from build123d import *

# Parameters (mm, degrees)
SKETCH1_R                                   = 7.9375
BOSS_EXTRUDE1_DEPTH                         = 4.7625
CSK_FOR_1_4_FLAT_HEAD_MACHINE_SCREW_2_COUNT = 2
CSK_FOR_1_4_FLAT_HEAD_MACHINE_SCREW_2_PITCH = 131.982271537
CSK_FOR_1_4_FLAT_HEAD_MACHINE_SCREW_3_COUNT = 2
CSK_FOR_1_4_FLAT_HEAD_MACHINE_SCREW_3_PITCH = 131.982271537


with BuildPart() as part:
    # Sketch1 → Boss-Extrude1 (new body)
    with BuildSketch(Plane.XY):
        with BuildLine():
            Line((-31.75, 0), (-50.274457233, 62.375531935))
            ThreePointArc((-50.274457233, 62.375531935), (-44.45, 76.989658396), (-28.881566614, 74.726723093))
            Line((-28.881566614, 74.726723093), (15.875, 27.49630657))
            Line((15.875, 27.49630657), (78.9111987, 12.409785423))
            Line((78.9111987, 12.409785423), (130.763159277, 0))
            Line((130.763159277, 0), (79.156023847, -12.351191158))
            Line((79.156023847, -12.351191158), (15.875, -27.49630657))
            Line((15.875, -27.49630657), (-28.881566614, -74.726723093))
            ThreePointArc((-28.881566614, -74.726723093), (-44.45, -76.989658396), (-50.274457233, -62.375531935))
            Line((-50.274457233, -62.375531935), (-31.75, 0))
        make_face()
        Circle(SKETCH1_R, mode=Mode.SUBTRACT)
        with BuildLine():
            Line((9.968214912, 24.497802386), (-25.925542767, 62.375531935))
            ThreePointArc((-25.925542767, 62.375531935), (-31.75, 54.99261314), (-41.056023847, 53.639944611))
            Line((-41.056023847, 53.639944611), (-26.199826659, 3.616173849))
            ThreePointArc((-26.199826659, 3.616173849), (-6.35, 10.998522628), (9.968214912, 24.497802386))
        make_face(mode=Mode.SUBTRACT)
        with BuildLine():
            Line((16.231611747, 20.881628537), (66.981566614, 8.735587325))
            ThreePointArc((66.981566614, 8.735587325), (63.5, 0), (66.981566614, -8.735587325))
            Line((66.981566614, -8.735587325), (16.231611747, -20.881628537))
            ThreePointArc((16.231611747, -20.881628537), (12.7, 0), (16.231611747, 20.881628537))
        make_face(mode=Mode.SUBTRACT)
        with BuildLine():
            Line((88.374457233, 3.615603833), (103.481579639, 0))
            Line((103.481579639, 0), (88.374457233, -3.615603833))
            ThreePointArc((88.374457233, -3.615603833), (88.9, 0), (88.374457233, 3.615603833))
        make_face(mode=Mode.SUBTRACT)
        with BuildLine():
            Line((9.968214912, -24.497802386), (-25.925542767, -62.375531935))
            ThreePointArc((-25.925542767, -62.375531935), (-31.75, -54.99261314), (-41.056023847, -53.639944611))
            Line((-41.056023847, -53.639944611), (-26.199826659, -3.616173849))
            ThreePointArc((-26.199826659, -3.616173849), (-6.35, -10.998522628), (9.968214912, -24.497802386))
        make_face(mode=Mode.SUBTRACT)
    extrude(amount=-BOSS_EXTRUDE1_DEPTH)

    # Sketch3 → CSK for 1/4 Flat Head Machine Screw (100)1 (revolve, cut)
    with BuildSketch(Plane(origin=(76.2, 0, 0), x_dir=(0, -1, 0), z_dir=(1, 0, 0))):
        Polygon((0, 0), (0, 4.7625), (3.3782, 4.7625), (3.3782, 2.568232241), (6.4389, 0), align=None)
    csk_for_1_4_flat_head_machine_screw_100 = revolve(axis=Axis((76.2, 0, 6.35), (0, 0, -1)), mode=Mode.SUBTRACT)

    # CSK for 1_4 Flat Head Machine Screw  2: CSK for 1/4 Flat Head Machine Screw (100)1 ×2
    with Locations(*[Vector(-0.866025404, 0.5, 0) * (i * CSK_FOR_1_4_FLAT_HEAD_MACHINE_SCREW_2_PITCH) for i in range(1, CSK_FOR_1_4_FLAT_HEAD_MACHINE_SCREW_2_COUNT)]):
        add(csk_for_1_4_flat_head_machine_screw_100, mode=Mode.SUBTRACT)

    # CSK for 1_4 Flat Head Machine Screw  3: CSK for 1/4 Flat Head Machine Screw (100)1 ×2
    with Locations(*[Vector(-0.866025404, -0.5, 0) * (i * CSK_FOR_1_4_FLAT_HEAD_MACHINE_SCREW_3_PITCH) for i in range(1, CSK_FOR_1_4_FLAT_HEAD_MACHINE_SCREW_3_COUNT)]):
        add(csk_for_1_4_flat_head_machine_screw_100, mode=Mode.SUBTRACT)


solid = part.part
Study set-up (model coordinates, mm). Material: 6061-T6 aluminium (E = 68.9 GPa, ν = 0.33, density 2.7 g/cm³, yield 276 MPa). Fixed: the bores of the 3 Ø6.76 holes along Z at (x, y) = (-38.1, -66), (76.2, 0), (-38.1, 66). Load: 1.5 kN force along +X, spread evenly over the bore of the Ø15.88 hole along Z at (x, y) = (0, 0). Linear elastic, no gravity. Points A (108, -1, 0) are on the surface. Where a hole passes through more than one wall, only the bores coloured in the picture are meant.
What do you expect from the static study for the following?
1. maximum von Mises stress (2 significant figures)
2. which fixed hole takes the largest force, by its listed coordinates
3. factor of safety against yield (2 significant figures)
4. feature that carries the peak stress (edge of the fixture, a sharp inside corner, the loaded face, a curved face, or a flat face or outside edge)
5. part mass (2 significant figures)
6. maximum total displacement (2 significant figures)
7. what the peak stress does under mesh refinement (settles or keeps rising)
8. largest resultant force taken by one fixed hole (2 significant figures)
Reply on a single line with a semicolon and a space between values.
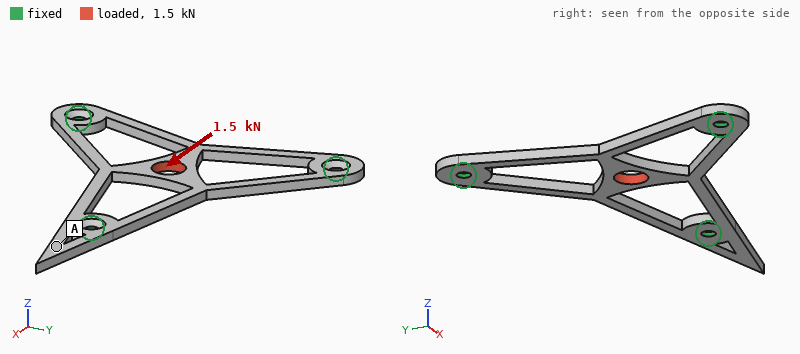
91 MPa; (76.2, 0); 3.0; a curved face; 61 g; 78 µm; settles; 1.1 kN
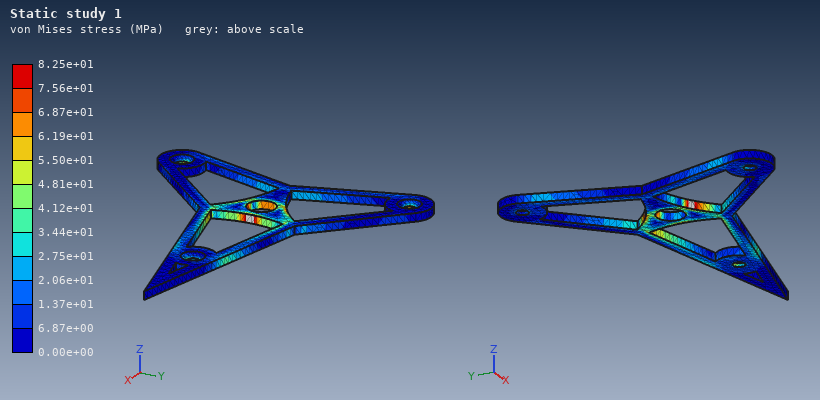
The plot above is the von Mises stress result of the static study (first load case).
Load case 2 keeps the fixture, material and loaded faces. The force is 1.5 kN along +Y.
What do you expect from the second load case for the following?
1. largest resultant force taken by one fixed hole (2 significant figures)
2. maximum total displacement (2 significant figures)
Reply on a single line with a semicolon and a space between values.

930 N; 74 µm
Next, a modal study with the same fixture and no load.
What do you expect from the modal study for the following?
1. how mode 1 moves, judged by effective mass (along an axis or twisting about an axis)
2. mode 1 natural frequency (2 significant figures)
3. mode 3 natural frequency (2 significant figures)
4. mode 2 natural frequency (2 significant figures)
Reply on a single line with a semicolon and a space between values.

along Z; 1000 Hz; 1900 Hz; 1900 Hz
